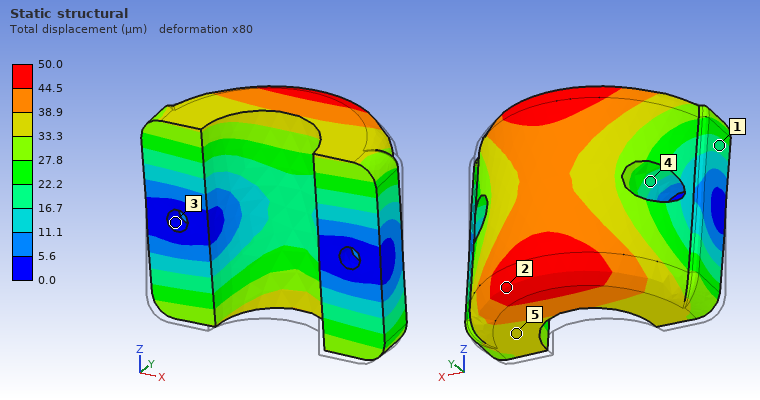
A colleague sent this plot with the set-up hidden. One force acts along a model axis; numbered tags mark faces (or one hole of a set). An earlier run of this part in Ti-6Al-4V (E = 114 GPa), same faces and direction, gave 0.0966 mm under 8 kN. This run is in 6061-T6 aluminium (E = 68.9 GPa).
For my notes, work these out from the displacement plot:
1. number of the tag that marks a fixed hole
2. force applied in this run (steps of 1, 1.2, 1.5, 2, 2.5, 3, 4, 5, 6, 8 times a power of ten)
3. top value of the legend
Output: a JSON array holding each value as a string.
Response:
["3", "2.5 kN", "50.0 µm"]
